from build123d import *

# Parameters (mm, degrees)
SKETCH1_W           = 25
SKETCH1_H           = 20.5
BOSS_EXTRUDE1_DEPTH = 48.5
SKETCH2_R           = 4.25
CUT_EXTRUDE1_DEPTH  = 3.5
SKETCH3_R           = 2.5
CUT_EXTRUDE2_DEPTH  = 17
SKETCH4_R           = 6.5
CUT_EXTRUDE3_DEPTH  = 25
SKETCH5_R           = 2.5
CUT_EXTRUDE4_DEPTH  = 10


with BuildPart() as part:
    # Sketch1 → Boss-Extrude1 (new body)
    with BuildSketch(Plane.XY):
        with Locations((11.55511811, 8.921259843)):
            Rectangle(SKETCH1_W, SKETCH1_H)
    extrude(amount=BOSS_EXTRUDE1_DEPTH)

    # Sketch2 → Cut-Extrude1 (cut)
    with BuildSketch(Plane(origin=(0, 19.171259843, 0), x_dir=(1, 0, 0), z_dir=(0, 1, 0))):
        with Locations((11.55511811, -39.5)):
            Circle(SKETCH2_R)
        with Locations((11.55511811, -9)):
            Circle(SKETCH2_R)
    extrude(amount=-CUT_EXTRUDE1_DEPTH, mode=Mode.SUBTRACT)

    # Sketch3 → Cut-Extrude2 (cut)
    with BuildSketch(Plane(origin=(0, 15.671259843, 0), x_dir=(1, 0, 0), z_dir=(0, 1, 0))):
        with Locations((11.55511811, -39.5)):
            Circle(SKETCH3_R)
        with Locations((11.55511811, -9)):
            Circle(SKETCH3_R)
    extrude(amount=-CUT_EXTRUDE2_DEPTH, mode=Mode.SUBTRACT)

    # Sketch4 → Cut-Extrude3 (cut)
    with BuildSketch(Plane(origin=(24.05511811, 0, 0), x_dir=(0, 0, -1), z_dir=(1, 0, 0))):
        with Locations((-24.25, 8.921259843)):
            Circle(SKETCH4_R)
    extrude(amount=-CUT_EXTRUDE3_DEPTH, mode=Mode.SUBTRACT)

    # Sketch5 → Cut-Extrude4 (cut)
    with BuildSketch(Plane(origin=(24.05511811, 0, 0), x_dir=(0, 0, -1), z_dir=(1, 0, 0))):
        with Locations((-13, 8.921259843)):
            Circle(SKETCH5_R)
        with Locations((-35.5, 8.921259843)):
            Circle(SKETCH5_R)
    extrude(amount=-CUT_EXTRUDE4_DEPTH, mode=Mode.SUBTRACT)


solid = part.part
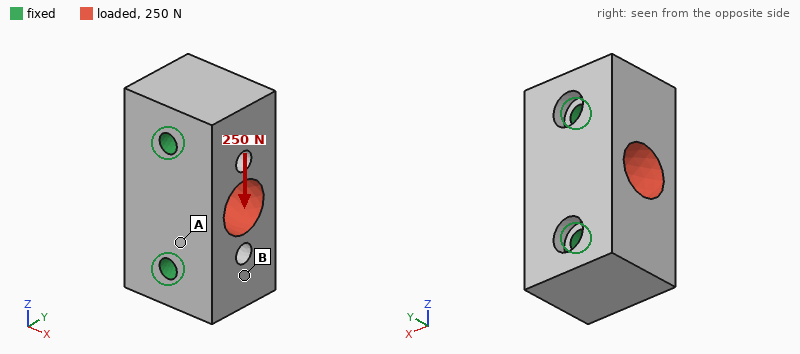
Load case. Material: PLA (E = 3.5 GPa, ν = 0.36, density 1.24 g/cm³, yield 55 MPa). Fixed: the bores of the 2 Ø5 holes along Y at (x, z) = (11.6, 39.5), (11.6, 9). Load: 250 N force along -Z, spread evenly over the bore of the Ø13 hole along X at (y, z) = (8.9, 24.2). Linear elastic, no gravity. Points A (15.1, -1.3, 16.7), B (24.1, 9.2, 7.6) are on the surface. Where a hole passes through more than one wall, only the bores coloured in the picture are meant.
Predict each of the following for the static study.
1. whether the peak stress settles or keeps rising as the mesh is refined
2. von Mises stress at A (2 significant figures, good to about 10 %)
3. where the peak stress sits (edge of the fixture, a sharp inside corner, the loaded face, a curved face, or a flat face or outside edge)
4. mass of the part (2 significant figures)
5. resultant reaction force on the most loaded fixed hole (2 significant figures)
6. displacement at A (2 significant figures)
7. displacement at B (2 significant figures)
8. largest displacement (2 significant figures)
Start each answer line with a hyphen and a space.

- keeps rising
- 0.30 MPa
- edge of the fixture
- 25 g
- 130 N
- 0.86 µm
- 1.1 µm
- 2.3 µm
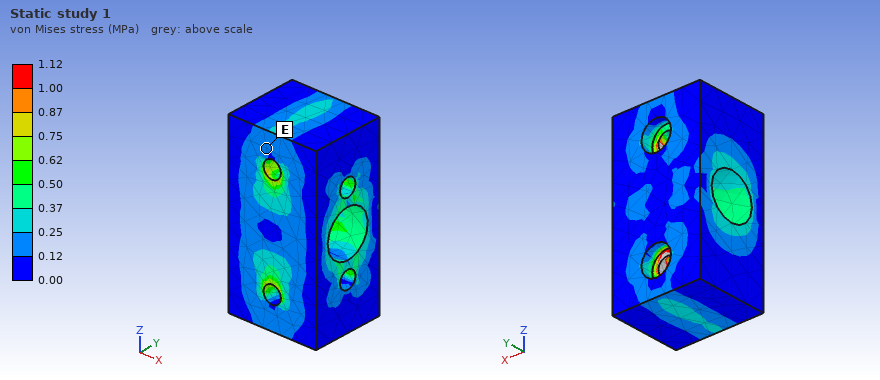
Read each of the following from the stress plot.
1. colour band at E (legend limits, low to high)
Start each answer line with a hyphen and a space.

- 0.12 to 0.25 MPa
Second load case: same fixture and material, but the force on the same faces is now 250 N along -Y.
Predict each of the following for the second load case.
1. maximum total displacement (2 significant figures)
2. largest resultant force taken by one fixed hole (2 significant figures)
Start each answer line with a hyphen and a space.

- 7.0 µm
- 130 N
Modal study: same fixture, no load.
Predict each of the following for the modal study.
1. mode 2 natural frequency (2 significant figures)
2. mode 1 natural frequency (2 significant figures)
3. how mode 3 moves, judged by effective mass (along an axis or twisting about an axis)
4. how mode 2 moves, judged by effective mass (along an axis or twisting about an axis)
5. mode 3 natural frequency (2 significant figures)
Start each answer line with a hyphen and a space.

- 11 kHz
- 10 kHz
- twisting about Y
- twisting about Z
- 12 kHz
